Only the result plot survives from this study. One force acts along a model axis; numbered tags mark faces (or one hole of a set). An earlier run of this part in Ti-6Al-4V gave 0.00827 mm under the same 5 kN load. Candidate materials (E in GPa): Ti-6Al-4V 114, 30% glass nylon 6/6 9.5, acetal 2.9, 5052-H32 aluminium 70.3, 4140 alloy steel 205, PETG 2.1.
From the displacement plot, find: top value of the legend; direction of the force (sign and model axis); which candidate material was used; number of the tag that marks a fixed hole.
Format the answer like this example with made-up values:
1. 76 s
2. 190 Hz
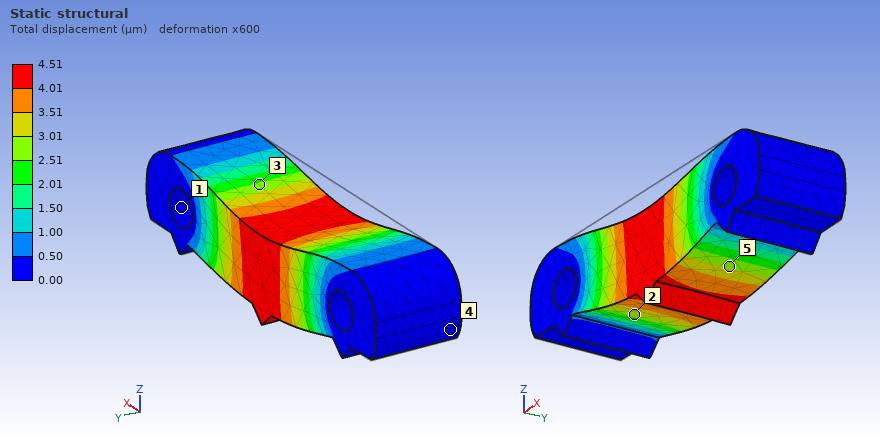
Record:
1. 4.51 µm
2. -Z
3. 4140 alloy steel
4. 1
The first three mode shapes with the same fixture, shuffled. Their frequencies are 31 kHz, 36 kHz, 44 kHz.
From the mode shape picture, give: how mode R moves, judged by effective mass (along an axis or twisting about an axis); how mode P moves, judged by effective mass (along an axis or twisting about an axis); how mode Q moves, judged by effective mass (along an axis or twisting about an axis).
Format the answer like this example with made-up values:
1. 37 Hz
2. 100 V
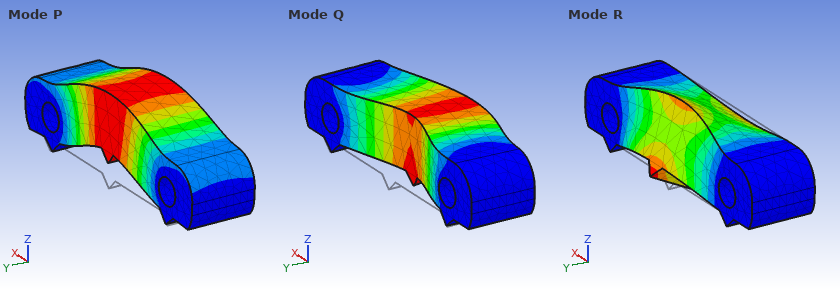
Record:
1. twisting about X
2. along Z
3. along Y
